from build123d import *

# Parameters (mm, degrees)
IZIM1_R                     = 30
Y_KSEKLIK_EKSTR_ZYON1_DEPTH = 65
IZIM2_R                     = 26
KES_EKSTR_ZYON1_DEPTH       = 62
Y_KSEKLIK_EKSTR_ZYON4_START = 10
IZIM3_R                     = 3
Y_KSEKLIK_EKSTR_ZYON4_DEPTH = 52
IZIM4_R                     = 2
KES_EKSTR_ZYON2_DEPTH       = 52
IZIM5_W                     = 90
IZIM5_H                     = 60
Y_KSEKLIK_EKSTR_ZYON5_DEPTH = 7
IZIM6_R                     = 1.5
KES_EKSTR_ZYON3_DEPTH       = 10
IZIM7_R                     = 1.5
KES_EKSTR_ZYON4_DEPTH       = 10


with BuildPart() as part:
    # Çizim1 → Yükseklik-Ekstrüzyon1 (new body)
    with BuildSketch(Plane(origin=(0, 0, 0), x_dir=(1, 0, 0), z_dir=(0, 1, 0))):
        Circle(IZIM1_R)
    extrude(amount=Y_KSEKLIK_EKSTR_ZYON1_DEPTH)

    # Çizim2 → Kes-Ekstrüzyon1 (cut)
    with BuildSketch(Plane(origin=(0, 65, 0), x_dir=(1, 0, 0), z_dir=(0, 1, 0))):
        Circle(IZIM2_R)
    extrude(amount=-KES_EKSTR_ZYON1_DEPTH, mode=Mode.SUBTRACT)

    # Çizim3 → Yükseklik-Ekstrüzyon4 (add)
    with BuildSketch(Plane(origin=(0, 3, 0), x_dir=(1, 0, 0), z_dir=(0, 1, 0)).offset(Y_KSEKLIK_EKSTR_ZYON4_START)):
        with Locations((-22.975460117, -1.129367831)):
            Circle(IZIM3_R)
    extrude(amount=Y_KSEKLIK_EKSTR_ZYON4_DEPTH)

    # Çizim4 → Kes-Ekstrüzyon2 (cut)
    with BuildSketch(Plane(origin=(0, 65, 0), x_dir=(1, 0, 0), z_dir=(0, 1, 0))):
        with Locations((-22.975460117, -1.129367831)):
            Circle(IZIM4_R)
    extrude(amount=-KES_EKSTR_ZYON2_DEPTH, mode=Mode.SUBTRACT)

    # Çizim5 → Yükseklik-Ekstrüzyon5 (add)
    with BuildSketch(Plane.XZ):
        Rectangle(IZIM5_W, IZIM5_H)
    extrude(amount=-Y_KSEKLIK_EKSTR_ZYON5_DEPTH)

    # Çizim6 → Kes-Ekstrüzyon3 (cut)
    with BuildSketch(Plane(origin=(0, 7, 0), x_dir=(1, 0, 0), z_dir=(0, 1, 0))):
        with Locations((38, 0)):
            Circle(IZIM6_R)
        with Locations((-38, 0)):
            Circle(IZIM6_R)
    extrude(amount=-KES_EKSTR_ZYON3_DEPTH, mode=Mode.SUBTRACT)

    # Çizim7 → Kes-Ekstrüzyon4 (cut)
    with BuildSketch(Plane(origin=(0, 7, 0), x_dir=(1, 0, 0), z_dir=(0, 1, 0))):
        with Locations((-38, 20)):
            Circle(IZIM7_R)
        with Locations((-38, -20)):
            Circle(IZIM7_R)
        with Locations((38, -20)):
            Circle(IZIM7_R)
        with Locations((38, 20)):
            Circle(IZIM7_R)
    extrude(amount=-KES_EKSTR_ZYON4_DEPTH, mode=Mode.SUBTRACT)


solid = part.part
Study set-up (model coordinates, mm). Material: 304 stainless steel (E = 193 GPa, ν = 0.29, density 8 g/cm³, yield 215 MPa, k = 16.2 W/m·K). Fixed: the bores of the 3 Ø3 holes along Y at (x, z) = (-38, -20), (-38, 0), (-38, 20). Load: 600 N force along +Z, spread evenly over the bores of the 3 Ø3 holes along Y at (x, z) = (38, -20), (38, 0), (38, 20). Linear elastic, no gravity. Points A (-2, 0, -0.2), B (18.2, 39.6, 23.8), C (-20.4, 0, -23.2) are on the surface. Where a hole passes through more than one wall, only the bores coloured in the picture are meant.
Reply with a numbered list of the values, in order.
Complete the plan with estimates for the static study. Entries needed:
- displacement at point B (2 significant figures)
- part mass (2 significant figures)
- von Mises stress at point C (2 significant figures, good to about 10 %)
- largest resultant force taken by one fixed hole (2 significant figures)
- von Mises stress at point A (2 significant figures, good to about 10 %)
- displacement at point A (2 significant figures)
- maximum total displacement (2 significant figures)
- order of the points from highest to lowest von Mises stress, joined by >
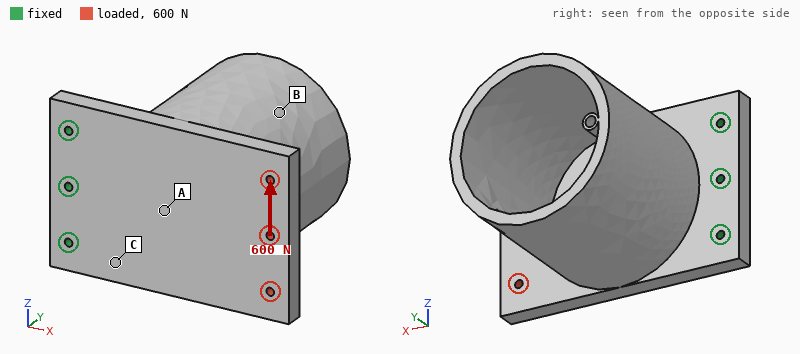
1. 4.3 µm
2. 630 g
3. 6.4 MPa
4. 1.1 kN
5. 4.1 MPa
6. 2.5 µm
7. 7.5 µm
8. C > A > B
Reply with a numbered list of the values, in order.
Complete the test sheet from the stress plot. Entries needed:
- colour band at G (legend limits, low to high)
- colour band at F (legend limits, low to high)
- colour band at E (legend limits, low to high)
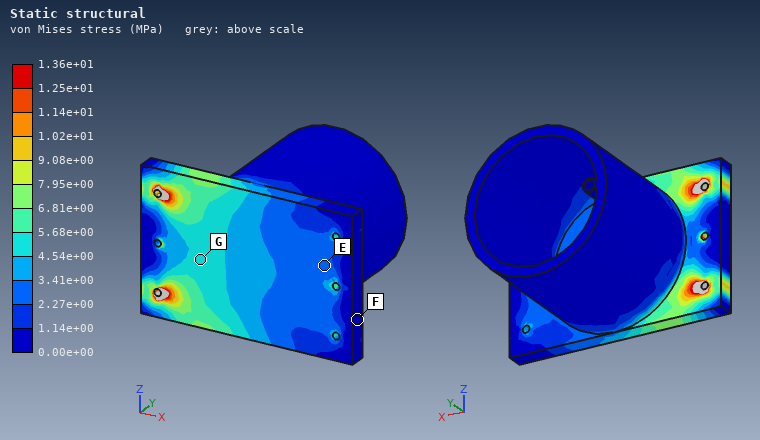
1. 4.54e+00 to 5.68e+00 MPa
2. 0.00e+00 to 1.14e+00 MPa
3. 2.27e+00 to 3.41e+00 MPa
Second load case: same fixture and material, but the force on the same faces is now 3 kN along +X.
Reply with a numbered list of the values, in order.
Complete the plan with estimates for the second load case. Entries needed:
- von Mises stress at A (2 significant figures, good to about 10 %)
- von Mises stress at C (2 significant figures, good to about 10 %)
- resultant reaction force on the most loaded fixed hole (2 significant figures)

1. 8.4 MPa
2. 7.4 MPa
3. 1.0 kN
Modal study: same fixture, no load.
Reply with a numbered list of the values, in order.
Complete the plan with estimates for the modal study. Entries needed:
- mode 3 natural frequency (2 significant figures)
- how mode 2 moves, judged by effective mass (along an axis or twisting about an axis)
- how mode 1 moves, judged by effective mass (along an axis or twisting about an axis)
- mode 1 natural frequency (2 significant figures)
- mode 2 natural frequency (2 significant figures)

1. 3600 Hz
2. along Z
3. along Y
4. 560 Hz
5. 1700 Hz
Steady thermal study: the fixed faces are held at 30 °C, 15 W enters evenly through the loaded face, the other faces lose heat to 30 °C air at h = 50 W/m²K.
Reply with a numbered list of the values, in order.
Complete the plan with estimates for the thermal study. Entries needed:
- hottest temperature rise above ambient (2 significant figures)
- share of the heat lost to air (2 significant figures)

1. 52 K
2. 93 %
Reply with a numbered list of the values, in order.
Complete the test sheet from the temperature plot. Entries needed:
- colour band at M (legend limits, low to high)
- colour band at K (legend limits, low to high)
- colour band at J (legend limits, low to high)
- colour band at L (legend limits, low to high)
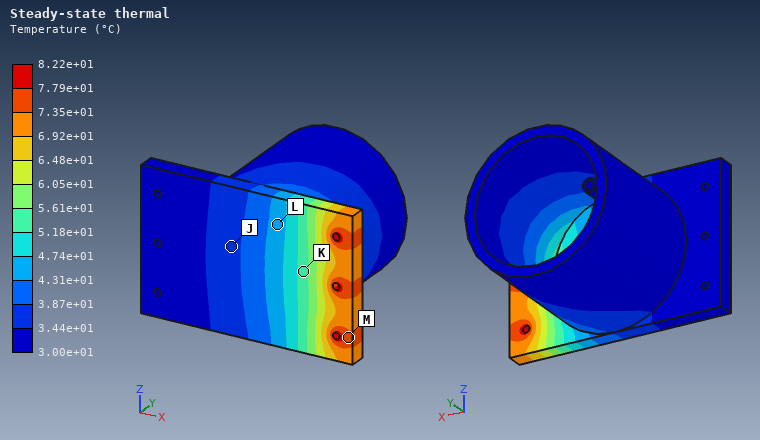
1. 7.35e+01 to 7.79e+01 °C
2. 5.18e+01 to 5.61e+01 °C
3. 3.44e+01 to 3.87e+01 °C
4. 4.31e+01 to 4.74e+01 °C
